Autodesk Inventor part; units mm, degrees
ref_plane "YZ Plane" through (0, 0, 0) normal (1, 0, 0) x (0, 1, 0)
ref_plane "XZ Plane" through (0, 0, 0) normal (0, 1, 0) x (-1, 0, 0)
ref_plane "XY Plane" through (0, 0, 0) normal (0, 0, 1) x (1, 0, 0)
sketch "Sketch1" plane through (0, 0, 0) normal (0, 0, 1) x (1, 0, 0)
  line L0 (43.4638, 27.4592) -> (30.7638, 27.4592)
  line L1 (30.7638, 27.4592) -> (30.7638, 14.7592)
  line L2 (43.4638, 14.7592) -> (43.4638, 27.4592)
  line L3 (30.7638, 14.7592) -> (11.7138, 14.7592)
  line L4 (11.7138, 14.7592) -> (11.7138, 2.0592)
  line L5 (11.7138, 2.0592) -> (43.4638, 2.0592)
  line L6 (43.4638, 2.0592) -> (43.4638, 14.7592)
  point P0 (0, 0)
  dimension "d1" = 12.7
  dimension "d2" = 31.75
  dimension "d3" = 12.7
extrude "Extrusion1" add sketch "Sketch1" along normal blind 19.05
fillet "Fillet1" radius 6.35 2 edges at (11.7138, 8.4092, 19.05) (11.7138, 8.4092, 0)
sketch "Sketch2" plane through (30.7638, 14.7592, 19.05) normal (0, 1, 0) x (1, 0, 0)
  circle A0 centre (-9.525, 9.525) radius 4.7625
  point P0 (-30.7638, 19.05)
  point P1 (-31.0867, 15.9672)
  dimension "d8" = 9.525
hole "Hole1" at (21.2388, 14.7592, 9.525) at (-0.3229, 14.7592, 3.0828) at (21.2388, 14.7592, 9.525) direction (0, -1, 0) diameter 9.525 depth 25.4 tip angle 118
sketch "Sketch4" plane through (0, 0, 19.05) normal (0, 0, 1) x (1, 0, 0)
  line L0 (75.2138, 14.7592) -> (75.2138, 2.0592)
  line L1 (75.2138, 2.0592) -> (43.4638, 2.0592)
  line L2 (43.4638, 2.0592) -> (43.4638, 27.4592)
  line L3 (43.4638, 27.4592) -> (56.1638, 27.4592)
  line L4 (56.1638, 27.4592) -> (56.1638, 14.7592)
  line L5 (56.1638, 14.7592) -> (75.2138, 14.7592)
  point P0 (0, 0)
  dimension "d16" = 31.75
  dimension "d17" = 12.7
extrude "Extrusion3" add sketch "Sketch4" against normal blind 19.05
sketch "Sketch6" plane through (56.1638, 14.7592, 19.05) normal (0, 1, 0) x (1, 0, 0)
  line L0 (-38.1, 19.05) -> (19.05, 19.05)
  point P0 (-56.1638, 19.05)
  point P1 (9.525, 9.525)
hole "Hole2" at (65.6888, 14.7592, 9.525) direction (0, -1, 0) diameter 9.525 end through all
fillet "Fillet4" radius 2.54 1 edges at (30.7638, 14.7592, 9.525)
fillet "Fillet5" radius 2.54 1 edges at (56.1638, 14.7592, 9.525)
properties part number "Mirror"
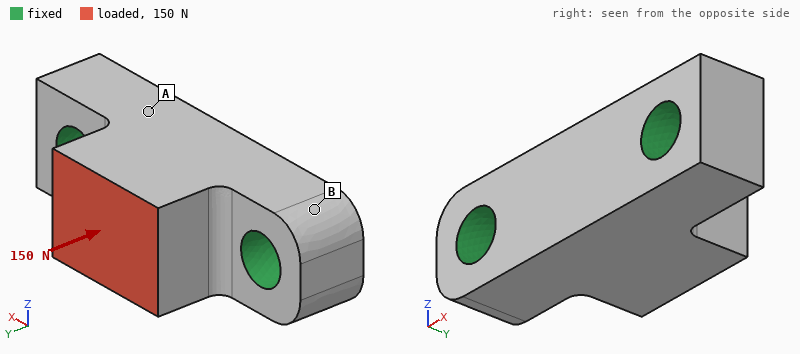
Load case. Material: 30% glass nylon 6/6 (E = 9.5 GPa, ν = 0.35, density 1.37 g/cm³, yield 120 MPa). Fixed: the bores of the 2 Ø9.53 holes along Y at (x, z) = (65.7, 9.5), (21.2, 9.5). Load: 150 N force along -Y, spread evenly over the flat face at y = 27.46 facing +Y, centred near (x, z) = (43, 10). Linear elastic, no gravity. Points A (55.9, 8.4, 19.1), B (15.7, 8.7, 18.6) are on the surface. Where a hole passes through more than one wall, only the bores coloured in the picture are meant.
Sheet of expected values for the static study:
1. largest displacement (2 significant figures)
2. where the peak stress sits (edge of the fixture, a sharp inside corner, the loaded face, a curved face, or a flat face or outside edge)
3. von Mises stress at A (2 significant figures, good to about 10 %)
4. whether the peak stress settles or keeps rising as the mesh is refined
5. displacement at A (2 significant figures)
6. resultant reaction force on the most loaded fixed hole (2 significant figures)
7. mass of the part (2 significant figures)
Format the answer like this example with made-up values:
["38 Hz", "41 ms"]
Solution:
["1.7 µm", "edge of the fixture", "0.49 MPa", "keeps rising", "0.86 µm", "80 N", "27 g"]
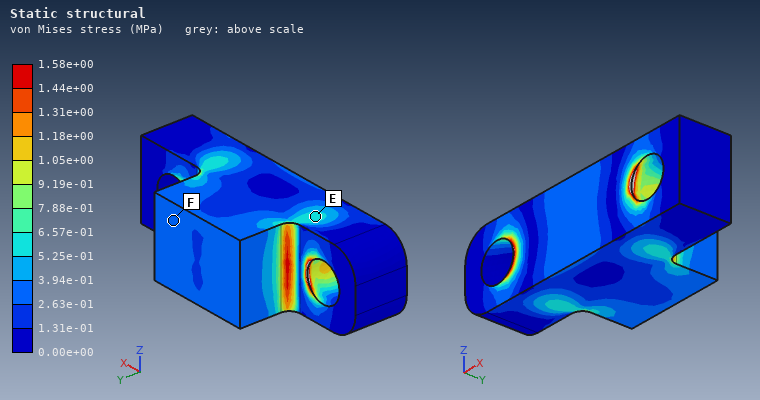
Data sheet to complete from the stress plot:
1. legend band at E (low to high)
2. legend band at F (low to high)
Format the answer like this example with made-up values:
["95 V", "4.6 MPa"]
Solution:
["5.25e-01 to 6.57e-01 MPa", "2.63e-01 to 3.94e-01 MPa"]
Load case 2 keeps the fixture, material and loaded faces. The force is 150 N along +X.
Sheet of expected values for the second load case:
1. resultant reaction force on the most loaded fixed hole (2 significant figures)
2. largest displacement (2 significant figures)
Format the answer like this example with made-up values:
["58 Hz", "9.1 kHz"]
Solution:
["110 N", "3.9 µm"]
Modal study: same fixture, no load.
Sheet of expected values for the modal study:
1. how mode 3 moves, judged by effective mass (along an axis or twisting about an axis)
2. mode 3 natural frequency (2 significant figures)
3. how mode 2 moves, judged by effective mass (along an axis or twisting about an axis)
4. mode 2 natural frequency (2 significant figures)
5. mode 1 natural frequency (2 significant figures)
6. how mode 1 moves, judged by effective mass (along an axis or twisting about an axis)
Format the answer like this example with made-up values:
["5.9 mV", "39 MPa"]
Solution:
["along Z", "16 kHz", "along Y", "13 kHz", "7500 Hz", "along Z"]
